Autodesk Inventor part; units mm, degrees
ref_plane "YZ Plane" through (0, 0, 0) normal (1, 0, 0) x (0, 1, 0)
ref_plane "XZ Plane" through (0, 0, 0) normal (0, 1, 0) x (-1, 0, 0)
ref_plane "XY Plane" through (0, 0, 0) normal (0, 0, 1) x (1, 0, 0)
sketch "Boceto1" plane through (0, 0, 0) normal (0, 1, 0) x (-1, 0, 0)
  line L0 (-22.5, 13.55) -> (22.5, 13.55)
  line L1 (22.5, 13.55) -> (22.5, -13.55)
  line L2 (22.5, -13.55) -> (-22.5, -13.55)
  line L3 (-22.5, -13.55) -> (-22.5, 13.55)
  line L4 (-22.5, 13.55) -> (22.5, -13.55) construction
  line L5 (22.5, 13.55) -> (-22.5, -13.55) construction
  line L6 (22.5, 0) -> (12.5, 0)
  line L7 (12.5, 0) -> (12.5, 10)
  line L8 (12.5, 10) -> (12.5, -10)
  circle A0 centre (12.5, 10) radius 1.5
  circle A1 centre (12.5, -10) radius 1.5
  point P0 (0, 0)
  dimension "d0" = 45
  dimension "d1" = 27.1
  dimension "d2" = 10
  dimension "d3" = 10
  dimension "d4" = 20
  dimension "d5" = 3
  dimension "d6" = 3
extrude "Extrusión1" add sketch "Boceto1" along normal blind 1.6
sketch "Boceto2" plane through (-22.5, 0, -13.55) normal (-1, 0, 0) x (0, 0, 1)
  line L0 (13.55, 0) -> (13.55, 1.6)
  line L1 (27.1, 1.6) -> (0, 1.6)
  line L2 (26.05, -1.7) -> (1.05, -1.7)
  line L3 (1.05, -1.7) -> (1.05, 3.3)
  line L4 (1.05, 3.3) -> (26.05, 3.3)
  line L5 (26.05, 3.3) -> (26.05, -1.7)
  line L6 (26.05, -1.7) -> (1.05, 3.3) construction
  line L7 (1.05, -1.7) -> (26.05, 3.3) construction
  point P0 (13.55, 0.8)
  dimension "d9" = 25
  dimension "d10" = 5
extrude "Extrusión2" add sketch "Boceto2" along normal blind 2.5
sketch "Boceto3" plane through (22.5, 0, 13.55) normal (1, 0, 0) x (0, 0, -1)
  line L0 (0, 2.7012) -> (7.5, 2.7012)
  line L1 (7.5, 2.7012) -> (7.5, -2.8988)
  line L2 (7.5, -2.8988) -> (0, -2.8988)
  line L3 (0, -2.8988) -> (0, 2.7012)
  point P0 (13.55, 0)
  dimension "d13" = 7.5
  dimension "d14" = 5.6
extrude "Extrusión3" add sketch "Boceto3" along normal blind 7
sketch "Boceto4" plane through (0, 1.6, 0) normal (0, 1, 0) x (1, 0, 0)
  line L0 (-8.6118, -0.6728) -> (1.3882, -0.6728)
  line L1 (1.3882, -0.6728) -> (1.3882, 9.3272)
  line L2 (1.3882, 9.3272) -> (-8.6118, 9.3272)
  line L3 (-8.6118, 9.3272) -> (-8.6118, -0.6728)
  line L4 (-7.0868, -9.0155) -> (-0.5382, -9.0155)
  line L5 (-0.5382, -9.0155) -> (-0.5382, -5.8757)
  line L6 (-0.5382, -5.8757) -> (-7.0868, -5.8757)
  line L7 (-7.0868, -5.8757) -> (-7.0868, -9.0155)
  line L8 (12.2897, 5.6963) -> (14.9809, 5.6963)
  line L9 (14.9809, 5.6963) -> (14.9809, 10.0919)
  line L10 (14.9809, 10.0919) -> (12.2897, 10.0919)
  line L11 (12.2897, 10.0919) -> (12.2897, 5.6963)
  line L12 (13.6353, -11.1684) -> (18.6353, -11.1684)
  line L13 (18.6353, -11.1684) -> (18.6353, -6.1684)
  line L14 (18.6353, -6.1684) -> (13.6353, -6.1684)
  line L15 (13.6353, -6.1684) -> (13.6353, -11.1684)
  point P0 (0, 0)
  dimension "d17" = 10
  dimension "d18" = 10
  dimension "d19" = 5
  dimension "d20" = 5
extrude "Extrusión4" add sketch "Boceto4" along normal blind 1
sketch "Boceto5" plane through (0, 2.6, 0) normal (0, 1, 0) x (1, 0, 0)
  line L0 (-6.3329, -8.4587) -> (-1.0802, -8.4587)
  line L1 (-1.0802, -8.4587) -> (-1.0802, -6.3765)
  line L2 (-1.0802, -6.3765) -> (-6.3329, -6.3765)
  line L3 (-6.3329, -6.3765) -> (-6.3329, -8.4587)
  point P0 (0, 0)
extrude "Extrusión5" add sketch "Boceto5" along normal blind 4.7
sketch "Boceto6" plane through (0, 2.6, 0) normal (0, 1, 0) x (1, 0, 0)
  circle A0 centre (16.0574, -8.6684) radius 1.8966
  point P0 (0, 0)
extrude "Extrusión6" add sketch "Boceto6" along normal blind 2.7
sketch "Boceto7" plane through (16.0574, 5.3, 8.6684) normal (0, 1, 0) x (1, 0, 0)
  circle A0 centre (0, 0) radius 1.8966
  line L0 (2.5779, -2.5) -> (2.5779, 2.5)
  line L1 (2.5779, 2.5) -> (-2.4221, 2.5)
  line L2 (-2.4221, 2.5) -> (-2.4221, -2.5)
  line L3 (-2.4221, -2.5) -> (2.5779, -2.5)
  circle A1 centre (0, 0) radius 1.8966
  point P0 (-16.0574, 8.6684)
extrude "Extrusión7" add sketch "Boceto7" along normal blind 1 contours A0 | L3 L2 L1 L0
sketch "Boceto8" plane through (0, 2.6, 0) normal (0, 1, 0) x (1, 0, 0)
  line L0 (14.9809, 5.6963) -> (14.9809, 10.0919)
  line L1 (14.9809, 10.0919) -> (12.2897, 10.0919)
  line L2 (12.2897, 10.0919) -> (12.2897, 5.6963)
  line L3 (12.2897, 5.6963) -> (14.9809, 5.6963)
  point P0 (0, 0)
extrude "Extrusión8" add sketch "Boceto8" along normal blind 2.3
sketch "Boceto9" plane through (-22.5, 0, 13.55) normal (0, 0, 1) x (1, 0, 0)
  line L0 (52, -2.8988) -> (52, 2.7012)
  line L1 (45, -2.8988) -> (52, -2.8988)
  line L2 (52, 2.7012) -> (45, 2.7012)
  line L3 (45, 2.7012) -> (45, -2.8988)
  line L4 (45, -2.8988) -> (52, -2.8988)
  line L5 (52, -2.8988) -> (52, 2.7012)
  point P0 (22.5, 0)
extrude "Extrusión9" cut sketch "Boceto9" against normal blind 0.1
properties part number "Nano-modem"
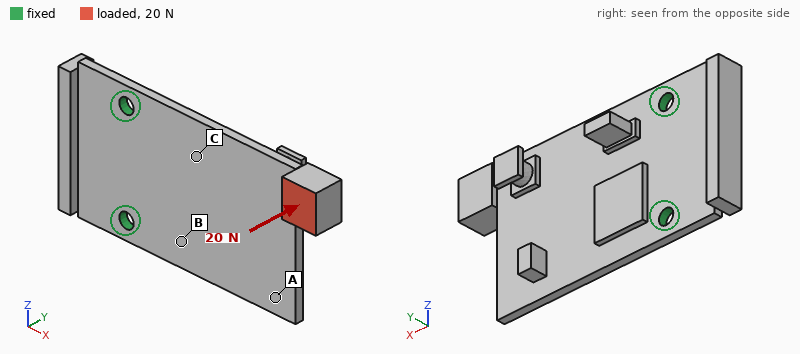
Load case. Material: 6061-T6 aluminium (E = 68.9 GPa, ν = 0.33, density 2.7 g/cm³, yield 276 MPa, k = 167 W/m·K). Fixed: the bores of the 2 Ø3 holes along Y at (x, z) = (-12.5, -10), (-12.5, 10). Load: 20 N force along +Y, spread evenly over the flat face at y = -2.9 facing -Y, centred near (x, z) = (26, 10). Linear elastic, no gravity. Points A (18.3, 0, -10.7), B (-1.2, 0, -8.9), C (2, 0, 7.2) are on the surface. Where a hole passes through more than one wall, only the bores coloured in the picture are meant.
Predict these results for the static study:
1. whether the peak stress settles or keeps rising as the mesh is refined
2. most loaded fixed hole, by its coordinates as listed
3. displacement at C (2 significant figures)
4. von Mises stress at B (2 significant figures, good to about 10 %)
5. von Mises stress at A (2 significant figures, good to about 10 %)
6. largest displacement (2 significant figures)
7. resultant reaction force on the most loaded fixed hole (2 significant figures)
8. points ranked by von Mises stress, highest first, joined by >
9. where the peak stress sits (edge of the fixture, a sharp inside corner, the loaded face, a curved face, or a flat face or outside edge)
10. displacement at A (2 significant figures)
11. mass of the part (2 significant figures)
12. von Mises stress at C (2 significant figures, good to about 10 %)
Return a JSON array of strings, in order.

["keeps rising", "(-12.5, 10)", "0.093 mm", "25 MPa", "11 MPa", "0.61 mm", "21 N", "C > B > A", "edge of the fixture", "0.26 mm", "7.6 g", "42 MPa"]
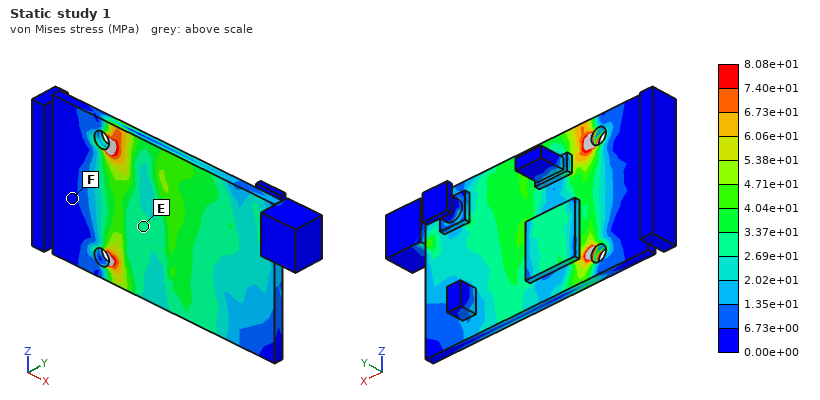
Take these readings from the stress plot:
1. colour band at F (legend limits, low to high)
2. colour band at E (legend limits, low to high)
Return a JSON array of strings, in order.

["0.00e+00 to 6.73e+00 MPa", "2.69e+01 to 3.37e+01 MPa"]
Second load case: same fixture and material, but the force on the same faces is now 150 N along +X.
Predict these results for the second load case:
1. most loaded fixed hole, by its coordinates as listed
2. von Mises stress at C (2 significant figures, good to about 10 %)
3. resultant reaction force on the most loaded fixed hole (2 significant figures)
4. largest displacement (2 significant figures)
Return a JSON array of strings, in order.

["(-12.5, 10)", "50 MPa", "150 N", "0.73 mm"]
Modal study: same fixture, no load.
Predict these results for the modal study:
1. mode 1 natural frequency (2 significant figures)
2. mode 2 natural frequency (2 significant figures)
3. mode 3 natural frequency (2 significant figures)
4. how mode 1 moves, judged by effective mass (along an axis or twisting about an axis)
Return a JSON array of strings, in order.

["820 Hz", "2800 Hz", "4800 Hz", "along Y"]
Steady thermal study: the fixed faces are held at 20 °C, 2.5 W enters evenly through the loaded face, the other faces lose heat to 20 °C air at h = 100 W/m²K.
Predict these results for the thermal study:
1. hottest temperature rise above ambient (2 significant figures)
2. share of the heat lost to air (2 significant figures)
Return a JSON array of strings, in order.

["14 K", "46 %"]
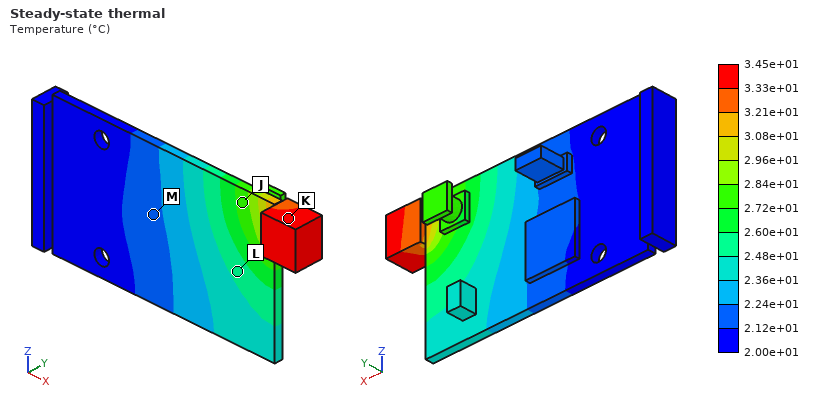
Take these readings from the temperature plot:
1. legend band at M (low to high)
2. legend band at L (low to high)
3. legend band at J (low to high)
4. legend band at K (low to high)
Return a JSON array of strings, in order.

["2.12e+01 to 2.24e+01 °C", "2.48e+01 to 2.60e+01 °C", "2.72e+01 to 2.84e+01 °C", "3.33e+01 to 3.45e+01 °C"]
